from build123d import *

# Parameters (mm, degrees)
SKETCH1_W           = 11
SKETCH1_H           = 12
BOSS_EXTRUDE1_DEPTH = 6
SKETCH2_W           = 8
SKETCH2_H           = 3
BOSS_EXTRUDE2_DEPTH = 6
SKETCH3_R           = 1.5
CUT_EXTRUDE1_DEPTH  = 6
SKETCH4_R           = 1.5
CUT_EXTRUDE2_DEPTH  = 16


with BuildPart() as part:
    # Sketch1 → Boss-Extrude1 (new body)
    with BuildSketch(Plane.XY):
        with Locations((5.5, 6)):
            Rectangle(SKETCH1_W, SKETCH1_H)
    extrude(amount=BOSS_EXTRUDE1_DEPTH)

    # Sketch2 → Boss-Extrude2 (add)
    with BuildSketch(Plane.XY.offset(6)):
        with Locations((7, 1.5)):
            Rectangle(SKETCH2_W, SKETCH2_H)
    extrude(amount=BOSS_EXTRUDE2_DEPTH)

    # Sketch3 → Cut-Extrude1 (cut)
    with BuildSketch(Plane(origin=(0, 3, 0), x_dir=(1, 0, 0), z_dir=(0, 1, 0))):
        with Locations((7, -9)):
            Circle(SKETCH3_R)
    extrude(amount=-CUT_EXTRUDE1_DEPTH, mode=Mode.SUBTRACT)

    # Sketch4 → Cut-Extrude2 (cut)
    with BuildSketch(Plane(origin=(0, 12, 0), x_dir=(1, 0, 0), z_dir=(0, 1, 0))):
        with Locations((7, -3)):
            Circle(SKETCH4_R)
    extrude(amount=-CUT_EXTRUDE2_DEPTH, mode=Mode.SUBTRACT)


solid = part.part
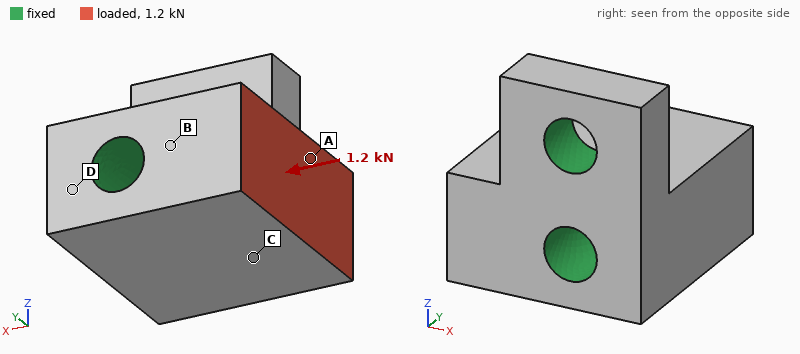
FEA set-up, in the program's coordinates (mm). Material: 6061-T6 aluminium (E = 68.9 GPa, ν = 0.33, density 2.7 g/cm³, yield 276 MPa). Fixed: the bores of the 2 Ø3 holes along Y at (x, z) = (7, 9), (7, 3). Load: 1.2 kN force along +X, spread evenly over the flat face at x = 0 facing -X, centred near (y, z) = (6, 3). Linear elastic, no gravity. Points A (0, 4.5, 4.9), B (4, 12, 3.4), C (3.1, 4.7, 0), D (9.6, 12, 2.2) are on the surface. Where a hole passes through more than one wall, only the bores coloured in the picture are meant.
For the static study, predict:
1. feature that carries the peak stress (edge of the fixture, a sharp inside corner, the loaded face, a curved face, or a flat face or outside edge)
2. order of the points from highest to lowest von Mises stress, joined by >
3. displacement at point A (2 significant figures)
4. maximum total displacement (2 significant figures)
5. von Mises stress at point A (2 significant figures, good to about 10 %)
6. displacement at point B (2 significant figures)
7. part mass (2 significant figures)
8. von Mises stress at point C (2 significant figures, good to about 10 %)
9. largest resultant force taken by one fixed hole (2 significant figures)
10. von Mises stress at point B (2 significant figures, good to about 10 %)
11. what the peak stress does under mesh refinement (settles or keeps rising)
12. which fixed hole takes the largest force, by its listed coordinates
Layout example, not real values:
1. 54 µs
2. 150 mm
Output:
1. edge of the fixture
2. B > A > C > D
3. 1.4 µm
4. 1.9 µm
5. 17 MPa
6. 0.66 µm
7. 2.2 g
8. 14 MPa
9. 1.2 kN
10. 21 MPa
11. keeps rising
12. (7, 3)
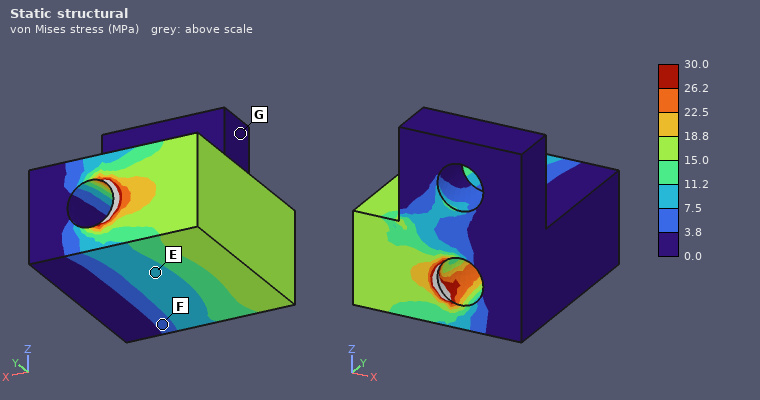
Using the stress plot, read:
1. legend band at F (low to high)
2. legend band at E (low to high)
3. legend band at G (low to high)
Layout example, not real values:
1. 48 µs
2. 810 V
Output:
1. 3.8 to 7.5 MPa
2. 7.5 to 11.2 MPa
3. 0.0 to 3.8 MPa
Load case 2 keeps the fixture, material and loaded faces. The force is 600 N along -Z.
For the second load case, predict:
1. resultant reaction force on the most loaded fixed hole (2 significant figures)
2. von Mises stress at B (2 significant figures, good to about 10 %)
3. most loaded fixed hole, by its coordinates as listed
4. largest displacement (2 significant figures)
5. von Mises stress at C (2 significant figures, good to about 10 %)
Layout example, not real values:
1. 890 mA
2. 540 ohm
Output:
1. 490 N
2. 23 MPa
3. (7, 3)
4. 7.7 µm
5. 24 MPa
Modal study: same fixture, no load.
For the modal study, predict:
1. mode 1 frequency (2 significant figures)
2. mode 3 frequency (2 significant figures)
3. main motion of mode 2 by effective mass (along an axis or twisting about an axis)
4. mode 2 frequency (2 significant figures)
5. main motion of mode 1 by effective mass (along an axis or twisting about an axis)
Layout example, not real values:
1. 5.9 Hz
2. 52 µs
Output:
1. 77 kHz
2. 110 kHz
3. along Y
4. 110 kHz
5. along Z
